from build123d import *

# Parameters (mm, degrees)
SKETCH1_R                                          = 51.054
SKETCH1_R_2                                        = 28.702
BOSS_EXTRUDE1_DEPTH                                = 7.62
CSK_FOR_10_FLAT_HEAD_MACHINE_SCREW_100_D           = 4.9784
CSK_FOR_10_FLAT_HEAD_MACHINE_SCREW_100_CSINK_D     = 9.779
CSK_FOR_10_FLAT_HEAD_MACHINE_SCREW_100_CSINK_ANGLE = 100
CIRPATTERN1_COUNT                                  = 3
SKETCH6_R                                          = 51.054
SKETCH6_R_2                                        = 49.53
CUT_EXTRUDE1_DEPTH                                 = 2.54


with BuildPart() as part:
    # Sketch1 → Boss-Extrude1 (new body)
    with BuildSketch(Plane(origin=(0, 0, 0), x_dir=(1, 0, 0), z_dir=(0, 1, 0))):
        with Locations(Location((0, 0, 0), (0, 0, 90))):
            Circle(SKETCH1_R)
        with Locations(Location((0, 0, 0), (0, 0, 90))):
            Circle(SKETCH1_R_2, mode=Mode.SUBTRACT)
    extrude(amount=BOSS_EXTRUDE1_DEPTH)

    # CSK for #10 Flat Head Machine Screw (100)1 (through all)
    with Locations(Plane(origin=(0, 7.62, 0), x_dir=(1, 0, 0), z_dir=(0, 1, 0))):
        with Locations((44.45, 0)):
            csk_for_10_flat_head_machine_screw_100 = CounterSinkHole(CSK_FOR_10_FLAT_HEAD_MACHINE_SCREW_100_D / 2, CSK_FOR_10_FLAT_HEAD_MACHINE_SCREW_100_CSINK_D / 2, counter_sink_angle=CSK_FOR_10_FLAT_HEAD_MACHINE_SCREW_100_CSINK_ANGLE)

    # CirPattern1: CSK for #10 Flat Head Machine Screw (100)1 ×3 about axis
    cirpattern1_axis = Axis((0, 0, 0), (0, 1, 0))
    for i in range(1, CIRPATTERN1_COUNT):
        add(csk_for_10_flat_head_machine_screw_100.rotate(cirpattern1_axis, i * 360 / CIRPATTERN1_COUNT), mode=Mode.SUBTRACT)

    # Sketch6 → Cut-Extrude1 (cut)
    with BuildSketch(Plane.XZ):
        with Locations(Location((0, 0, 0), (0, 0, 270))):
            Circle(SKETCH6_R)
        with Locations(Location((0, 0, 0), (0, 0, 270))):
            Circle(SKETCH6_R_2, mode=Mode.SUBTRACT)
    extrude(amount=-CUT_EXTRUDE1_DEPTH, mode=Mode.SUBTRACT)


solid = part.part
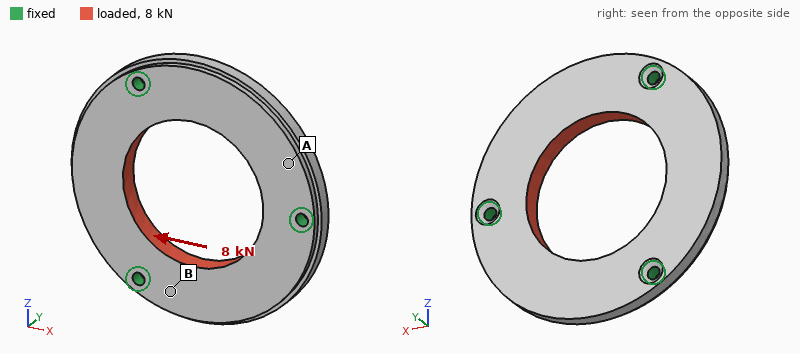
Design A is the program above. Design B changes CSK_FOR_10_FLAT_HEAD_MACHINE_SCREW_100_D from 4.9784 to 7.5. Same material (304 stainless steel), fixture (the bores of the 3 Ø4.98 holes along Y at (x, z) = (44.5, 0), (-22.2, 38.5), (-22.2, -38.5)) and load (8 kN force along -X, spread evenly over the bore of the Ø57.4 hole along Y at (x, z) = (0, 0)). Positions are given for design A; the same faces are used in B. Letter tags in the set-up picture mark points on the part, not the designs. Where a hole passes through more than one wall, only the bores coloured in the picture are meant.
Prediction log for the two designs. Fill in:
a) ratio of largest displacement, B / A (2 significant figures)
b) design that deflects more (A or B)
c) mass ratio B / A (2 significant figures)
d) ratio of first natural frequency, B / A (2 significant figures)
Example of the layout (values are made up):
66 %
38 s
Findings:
0.82
A
0.99
1.2
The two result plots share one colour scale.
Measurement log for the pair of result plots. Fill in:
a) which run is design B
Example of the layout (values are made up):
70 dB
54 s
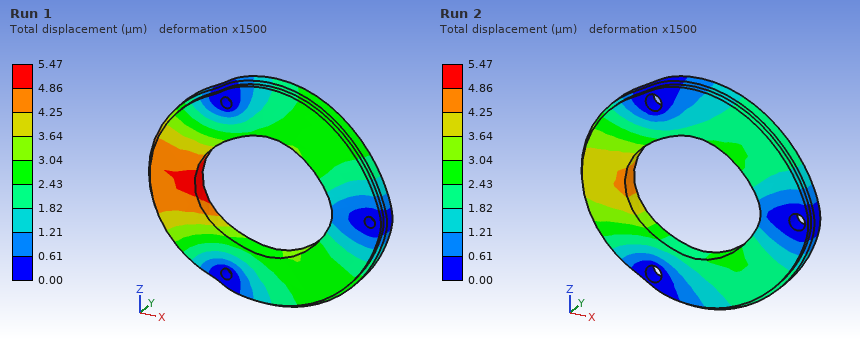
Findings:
Run 2
